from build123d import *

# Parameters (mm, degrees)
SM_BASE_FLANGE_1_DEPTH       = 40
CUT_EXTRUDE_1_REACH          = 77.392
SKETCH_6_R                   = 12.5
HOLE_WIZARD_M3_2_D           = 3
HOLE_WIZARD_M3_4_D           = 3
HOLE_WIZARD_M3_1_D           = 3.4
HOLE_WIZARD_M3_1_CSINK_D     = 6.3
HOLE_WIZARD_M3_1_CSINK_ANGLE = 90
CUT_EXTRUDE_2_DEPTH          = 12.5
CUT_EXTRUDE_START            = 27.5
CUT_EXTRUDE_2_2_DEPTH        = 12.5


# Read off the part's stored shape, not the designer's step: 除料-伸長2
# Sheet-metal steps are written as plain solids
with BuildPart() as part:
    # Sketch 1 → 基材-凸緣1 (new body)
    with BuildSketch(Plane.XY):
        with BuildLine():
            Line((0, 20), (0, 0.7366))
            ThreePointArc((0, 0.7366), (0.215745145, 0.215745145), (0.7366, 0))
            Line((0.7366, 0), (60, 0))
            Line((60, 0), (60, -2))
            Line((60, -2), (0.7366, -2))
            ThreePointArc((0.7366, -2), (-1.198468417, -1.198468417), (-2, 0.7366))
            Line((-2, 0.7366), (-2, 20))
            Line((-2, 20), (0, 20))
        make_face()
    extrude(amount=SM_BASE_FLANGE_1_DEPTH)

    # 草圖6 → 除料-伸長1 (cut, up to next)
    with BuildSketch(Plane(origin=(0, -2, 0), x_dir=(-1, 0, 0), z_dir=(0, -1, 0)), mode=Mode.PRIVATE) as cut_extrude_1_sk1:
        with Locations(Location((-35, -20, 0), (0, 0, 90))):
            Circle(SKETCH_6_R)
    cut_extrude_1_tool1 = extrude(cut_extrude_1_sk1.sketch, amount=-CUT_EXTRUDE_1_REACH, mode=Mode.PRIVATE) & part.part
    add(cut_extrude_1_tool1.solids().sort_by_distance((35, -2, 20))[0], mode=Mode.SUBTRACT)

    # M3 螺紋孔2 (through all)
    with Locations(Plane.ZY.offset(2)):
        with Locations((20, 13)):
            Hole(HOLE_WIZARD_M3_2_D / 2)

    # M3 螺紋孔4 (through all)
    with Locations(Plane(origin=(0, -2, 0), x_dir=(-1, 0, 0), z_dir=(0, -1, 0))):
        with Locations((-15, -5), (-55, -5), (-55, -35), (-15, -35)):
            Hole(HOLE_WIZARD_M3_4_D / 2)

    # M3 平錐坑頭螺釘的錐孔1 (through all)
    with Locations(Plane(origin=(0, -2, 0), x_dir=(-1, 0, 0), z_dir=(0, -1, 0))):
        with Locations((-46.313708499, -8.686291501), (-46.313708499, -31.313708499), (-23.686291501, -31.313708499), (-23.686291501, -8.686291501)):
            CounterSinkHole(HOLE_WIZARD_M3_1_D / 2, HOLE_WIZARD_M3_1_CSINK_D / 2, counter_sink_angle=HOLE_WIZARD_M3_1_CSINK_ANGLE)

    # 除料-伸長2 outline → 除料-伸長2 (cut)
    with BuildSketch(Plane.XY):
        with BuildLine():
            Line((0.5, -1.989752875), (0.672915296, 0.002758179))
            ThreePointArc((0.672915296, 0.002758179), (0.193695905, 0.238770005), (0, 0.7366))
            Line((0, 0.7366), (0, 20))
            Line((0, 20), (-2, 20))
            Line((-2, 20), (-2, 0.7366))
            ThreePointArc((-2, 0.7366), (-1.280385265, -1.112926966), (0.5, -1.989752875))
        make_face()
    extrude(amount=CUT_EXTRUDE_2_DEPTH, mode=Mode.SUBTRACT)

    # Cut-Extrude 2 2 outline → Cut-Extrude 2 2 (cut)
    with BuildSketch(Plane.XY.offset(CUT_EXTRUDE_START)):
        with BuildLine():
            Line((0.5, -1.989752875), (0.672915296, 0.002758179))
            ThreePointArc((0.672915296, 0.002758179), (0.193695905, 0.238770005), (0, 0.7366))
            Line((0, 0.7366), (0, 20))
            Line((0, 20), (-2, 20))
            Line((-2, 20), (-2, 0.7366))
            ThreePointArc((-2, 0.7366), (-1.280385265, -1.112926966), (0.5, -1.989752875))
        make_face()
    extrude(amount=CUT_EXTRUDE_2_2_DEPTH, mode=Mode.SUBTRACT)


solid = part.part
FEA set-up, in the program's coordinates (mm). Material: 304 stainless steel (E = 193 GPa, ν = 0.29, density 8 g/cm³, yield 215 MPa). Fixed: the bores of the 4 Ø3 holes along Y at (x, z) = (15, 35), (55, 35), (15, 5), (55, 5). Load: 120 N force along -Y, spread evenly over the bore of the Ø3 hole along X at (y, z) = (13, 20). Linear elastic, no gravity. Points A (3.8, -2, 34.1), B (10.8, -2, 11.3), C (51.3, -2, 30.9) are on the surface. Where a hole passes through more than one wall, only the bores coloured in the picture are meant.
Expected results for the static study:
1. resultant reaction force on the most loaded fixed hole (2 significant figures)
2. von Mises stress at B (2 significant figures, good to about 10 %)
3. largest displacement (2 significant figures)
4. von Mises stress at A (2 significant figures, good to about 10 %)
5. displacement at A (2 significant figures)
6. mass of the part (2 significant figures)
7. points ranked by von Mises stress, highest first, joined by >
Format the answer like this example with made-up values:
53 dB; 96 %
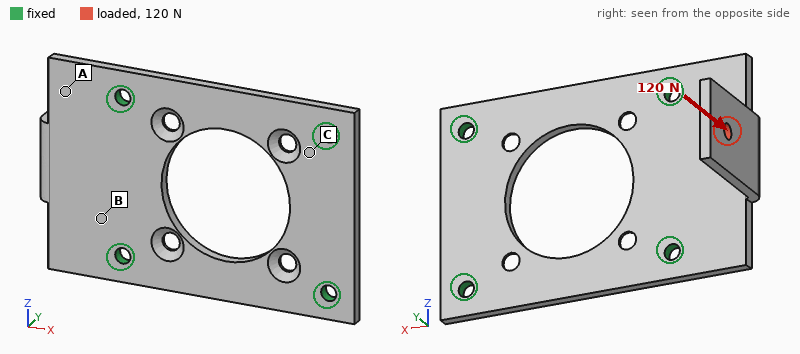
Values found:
63 N; 51 MPa; 0.10 mm; 31 MPa; 0.021 mm; 34 g; B > A > C
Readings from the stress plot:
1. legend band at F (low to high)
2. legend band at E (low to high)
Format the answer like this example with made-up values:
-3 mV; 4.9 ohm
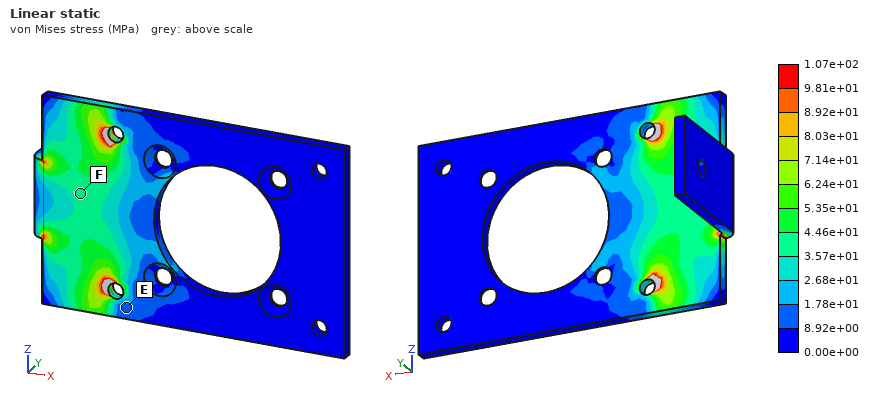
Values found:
3.57e+01 to 4.46e+01 MPa; 8.92e+00 to 1.78e+01 MPa
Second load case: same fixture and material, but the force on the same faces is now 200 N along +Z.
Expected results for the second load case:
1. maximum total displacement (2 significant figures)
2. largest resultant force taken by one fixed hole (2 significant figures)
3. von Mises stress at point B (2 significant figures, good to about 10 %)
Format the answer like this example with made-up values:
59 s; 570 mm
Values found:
0.12 mm; 180 N; 57 MPa
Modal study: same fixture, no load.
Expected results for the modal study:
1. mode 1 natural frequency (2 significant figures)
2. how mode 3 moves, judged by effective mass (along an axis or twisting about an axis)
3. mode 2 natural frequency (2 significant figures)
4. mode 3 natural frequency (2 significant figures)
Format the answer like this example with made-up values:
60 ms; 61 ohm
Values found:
2000 Hz; along Y; 3900 Hz; 4300 Hz
